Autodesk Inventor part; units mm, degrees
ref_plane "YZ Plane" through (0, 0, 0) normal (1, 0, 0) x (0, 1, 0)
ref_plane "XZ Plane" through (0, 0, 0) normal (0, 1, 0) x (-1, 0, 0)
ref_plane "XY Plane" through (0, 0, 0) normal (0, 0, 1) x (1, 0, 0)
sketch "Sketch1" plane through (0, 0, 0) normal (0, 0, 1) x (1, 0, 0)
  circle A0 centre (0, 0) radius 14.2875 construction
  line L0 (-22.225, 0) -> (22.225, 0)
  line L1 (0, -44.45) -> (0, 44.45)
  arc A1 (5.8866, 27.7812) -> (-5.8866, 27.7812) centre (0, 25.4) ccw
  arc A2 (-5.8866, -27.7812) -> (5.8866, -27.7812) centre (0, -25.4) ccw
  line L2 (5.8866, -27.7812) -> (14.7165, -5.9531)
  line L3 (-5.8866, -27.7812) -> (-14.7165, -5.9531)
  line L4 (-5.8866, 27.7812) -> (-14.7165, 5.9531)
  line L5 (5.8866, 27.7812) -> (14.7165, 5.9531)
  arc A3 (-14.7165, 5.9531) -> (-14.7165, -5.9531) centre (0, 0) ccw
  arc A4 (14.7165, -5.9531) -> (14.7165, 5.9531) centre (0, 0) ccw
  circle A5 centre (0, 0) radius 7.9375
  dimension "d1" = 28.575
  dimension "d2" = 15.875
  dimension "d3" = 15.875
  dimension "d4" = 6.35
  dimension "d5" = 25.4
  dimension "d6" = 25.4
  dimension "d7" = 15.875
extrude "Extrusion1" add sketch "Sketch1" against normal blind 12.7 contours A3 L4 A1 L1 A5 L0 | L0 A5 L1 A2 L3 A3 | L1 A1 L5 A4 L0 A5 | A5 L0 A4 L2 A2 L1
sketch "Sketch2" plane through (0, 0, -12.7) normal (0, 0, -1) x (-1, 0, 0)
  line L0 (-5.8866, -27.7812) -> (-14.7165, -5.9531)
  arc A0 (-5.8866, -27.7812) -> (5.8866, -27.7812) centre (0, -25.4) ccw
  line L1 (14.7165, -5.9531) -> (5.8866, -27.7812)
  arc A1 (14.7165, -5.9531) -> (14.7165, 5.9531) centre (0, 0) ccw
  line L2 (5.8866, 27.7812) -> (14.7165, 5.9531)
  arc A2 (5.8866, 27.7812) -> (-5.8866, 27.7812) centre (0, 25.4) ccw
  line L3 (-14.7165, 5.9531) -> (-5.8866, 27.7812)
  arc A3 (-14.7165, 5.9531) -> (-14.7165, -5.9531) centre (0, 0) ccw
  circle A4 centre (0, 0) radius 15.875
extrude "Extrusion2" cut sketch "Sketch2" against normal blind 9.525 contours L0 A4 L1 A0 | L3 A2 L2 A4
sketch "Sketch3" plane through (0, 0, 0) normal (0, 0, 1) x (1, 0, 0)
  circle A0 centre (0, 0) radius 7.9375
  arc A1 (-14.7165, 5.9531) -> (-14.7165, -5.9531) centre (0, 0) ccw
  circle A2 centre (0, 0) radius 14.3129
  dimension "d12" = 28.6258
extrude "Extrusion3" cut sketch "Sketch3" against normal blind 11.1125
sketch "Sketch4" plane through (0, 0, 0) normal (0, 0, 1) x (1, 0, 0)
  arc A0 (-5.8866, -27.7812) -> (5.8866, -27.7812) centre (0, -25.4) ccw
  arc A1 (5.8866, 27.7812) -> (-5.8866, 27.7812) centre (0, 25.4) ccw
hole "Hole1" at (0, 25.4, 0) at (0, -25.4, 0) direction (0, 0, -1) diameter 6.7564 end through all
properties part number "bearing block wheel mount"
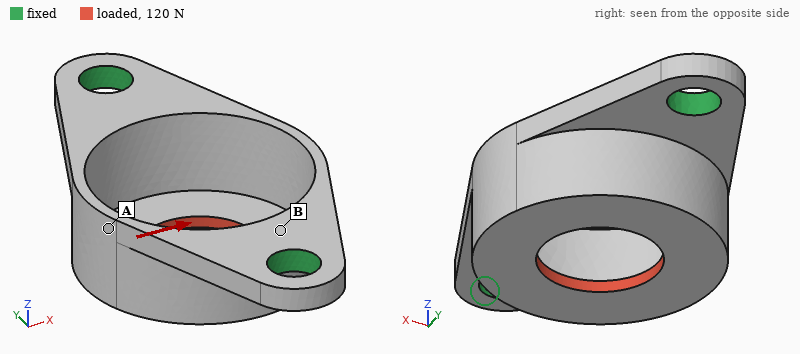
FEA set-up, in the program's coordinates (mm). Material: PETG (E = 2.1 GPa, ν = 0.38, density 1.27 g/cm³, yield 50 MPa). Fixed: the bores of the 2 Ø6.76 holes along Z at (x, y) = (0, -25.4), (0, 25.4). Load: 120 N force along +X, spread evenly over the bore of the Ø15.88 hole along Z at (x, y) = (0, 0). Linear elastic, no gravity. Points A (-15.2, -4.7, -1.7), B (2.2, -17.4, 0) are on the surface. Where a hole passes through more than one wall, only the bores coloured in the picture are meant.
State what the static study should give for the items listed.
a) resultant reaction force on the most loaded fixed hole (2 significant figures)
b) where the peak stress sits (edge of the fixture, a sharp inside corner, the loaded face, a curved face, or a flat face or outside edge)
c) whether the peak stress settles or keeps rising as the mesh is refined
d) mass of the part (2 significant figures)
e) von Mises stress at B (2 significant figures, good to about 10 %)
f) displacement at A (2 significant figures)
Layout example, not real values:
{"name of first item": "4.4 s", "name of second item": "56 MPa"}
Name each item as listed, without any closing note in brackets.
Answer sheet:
{"resultant reaction force on the most loaded fixed hole": "60 N", "where the peak stress sits": "edge of the fixture", "whether the peak stress settles or keeps rising as the mesh is refined": "keeps rising", "mass of the part": "5.2 g", "von Mises stress at B": "11 MPa", "displacement at A": "0.54 mm"}
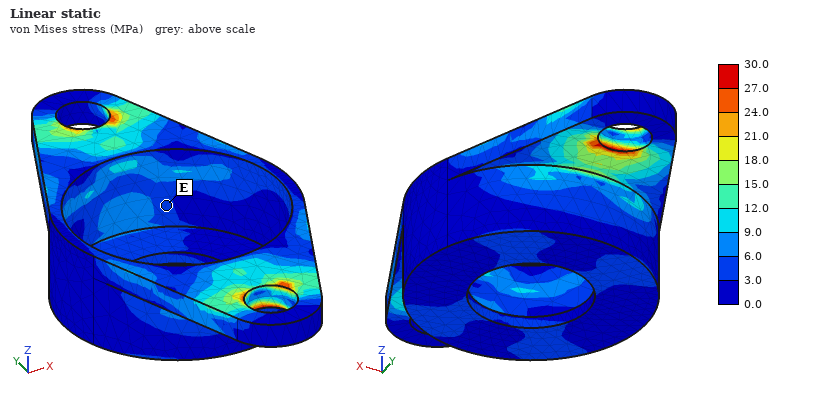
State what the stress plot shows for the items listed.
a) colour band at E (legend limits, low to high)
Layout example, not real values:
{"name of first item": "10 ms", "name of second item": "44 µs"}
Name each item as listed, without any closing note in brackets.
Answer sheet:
{"colour band at E": "3.0 to 6.0 MPa"}
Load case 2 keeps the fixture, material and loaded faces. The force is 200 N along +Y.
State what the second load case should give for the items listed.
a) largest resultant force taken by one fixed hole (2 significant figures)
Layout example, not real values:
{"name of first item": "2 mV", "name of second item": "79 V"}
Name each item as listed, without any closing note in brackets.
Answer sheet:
{"largest resultant force taken by one fixed hole": "110 N"}
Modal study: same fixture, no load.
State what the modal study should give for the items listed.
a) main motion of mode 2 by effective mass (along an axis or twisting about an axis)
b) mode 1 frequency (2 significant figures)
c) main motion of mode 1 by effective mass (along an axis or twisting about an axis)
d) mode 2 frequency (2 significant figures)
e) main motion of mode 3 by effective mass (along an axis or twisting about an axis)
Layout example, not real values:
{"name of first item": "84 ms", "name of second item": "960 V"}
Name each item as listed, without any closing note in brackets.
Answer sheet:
{"main motion of mode 2 by effective mass": "along Z", "mode 1 frequency": "1300 Hz", "main motion of mode 1 by effective mass": "along X", "mode 2 frequency": "2600 Hz", "main motion of mode 3 by effective mass": "along Y"}
